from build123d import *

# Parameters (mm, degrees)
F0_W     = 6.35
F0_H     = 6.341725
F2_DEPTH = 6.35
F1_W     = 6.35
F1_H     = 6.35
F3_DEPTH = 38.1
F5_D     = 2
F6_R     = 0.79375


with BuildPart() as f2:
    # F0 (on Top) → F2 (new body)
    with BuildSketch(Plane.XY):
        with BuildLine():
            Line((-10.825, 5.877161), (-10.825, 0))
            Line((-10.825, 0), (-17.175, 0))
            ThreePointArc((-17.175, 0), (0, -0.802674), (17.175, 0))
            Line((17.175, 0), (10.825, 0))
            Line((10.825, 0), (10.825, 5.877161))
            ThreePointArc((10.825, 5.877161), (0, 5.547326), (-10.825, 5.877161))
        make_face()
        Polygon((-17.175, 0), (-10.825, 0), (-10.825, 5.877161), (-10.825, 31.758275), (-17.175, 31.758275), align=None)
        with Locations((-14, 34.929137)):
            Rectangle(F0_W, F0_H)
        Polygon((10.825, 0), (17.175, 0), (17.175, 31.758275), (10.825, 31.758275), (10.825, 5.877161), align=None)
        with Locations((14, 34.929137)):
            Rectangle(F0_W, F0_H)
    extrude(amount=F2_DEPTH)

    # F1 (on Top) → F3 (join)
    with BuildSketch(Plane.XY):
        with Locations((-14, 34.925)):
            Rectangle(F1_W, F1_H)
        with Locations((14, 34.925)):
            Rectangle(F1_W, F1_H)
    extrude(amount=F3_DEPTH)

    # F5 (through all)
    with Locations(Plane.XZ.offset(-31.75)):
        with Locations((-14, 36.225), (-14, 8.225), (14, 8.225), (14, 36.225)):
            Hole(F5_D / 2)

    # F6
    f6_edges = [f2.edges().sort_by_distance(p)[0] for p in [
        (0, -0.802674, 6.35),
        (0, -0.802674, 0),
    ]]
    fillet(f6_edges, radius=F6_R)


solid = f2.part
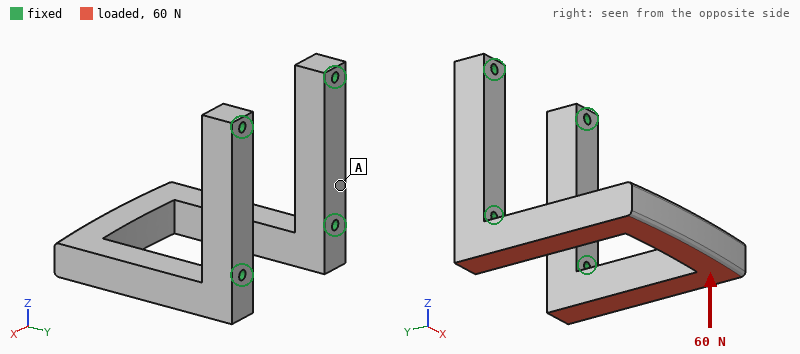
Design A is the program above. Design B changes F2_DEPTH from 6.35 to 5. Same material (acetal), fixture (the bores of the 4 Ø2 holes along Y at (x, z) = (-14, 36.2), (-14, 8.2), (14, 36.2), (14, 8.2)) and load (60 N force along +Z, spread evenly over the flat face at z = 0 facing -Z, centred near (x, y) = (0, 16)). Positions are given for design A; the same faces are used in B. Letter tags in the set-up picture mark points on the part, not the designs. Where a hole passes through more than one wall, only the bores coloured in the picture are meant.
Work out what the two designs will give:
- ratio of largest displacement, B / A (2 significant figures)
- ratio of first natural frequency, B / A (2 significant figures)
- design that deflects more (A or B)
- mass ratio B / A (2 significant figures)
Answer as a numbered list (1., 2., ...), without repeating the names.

1. 1.8
2. 0.85
3. B
4. 0.89
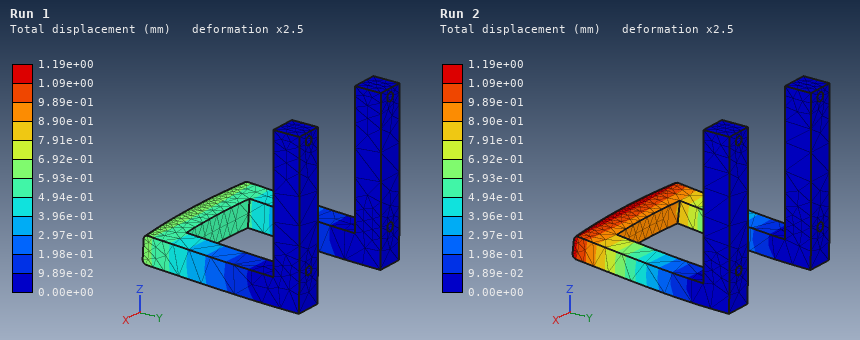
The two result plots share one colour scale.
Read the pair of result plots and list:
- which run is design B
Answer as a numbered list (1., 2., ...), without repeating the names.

1. Run 2
